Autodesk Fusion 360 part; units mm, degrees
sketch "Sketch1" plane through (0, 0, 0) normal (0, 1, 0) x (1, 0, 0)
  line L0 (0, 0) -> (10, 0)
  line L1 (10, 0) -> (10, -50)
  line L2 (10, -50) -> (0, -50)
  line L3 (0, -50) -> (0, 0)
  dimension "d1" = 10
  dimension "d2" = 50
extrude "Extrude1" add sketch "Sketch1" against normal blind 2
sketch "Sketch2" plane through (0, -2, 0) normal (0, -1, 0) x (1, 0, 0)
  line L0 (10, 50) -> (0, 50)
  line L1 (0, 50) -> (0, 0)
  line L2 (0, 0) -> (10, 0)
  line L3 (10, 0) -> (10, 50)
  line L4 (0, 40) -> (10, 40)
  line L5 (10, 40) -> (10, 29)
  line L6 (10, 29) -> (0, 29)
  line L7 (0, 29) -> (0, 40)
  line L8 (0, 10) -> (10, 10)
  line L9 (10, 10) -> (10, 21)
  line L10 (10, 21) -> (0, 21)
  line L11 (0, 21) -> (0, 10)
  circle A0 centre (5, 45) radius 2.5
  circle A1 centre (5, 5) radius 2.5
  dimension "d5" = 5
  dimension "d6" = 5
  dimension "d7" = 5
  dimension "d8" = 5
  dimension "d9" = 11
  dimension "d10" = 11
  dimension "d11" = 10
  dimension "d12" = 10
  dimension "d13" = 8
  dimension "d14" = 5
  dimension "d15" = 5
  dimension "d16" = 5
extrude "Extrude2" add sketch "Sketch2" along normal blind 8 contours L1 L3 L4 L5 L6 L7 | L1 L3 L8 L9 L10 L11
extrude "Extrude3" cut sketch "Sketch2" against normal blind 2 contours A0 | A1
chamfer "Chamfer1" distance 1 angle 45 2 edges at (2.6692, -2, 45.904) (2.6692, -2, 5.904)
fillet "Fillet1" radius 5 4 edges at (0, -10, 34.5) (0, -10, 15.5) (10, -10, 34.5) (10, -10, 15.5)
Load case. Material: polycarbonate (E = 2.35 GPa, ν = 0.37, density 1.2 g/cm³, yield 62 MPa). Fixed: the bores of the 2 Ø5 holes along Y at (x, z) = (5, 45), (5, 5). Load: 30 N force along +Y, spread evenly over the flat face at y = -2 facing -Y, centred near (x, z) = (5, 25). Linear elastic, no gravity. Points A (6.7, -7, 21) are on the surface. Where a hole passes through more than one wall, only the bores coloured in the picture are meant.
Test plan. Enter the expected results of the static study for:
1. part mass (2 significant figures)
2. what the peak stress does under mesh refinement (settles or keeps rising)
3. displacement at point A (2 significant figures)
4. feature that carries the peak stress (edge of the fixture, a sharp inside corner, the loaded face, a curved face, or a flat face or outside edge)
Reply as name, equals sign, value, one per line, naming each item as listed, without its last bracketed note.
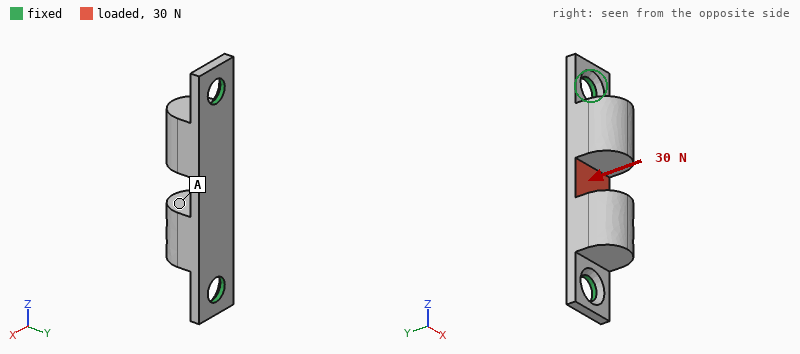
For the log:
part mass = 2.9 g
what the peak stress does under mesh refinement = keeps rising
displacement at point A = 0.46 mm
feature that carries the peak stress = edge of the fixture
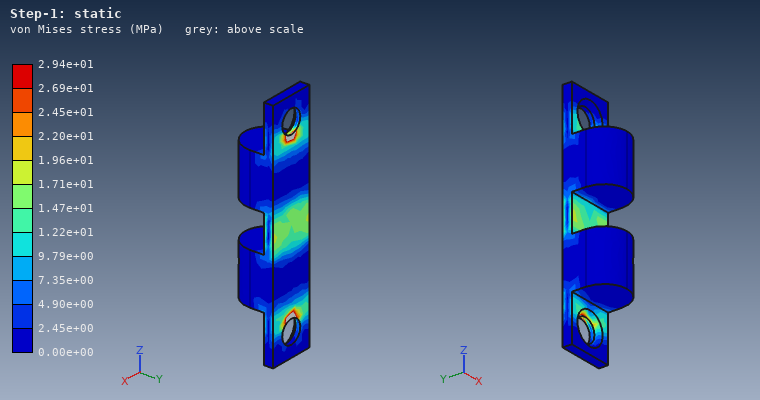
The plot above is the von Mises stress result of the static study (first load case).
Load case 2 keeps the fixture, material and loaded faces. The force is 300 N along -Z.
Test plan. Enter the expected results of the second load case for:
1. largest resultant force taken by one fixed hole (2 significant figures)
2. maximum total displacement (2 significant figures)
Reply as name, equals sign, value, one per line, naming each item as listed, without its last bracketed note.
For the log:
largest resultant force taken by one fixed hole = 150 N
maximum total displacement = 59 µm
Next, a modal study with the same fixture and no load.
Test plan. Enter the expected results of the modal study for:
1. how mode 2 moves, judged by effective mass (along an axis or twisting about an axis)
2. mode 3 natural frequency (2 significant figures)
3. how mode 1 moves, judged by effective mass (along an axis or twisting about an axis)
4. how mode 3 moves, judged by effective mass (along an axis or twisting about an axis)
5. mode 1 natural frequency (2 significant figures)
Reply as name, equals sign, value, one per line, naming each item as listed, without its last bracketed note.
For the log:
how mode 2 moves, judged by effective mass = along X
mode 3 natural frequency = 3100 Hz
how mode 1 moves, judged by effective mass = along Y
how mode 3 moves, judged by effective mass = twisting about Y
mode 1 natural frequency = 1200 Hz
